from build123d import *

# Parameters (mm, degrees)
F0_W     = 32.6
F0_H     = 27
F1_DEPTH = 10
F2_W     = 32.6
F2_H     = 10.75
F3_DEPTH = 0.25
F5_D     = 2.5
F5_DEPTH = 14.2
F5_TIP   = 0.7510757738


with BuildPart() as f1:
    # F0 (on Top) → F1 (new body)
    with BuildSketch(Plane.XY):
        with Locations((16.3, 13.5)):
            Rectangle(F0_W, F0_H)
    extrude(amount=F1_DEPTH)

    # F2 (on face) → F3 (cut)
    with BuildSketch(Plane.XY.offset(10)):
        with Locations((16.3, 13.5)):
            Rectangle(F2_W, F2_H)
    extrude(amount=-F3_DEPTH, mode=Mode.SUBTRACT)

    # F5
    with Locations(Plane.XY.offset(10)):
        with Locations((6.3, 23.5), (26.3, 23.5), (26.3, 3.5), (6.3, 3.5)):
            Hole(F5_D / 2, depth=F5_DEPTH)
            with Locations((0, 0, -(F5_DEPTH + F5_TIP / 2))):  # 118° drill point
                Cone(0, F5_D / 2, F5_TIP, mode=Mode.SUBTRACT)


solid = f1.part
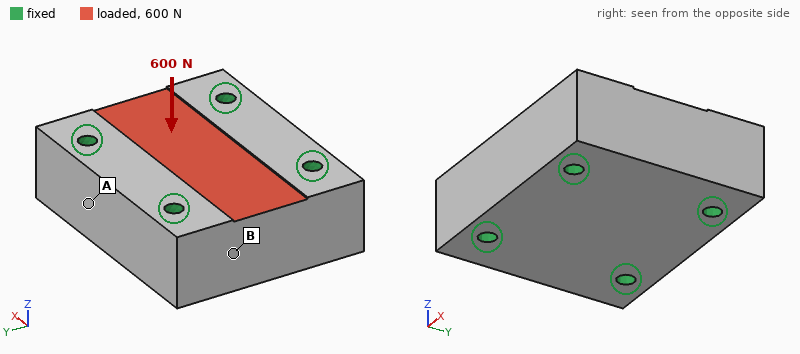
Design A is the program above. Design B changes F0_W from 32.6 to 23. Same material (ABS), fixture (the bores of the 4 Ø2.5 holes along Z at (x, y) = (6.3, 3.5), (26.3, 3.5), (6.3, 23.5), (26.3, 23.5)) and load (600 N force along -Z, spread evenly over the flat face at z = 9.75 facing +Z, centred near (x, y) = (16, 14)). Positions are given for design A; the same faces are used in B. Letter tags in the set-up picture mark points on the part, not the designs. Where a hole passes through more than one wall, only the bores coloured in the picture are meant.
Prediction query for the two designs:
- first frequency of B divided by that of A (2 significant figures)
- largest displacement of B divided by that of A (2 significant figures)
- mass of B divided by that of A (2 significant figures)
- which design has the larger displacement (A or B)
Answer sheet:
0.98
1.4
0.70
B
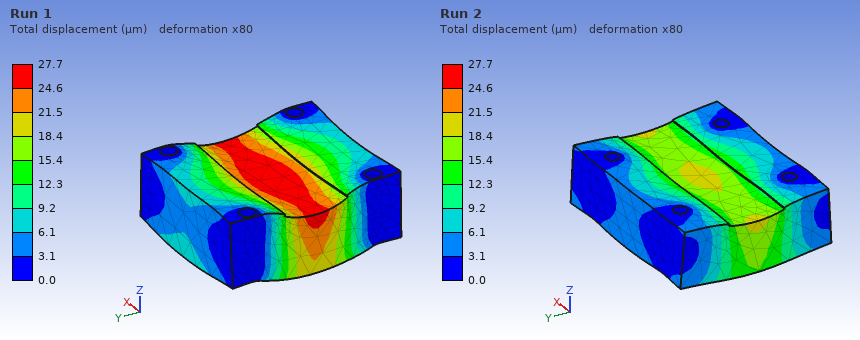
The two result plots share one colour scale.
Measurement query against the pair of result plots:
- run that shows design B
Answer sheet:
Run 1
